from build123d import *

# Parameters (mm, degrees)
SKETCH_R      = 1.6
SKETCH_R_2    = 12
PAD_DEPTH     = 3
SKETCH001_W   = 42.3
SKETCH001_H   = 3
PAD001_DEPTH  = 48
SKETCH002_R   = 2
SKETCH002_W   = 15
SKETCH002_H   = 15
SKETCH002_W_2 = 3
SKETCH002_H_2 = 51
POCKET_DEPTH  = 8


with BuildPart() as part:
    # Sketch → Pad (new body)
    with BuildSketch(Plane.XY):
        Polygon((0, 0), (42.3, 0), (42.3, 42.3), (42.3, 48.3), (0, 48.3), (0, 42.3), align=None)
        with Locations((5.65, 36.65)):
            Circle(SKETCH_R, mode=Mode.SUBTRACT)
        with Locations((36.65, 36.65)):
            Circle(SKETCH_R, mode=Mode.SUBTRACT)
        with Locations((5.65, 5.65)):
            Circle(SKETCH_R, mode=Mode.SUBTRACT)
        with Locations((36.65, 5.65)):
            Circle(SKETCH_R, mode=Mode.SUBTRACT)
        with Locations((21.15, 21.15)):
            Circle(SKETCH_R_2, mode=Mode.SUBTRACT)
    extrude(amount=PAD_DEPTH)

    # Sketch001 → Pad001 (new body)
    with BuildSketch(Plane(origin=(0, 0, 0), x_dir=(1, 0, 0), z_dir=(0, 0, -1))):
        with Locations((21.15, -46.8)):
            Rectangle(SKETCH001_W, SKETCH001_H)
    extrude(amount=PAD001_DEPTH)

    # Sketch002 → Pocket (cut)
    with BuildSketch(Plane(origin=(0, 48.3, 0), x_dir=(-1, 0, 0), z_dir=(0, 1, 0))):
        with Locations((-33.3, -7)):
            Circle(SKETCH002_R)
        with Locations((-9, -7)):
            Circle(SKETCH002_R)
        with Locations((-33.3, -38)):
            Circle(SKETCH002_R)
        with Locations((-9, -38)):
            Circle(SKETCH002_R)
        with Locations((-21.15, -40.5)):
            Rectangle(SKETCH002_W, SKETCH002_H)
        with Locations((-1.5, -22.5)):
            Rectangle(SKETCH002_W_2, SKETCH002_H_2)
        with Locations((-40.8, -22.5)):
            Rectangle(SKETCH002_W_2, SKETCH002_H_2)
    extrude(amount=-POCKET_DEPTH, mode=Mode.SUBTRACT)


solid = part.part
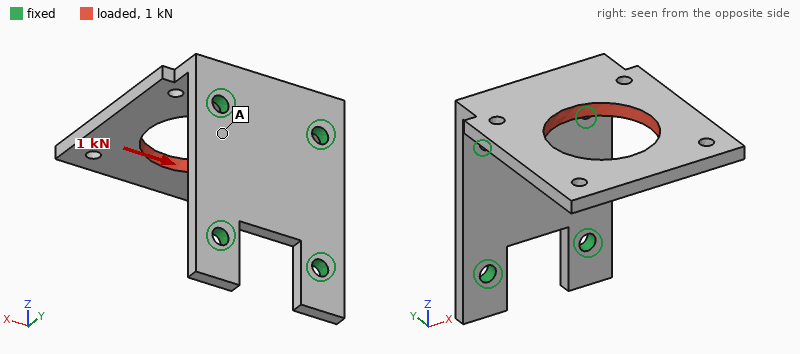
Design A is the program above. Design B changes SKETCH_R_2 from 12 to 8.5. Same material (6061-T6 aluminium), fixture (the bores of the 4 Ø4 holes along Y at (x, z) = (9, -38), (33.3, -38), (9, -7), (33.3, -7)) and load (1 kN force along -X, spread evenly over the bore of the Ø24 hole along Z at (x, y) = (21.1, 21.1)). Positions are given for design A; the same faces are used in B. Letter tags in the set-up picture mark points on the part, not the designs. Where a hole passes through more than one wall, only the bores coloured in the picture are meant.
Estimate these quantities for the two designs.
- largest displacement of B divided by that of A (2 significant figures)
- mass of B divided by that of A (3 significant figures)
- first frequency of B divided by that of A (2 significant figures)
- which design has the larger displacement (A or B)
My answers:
0.90
1.08
1.0
A
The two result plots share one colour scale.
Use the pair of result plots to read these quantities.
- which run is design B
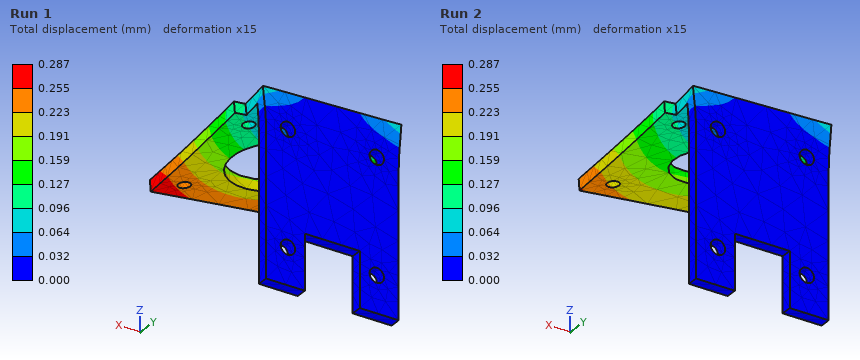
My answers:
Run 2
